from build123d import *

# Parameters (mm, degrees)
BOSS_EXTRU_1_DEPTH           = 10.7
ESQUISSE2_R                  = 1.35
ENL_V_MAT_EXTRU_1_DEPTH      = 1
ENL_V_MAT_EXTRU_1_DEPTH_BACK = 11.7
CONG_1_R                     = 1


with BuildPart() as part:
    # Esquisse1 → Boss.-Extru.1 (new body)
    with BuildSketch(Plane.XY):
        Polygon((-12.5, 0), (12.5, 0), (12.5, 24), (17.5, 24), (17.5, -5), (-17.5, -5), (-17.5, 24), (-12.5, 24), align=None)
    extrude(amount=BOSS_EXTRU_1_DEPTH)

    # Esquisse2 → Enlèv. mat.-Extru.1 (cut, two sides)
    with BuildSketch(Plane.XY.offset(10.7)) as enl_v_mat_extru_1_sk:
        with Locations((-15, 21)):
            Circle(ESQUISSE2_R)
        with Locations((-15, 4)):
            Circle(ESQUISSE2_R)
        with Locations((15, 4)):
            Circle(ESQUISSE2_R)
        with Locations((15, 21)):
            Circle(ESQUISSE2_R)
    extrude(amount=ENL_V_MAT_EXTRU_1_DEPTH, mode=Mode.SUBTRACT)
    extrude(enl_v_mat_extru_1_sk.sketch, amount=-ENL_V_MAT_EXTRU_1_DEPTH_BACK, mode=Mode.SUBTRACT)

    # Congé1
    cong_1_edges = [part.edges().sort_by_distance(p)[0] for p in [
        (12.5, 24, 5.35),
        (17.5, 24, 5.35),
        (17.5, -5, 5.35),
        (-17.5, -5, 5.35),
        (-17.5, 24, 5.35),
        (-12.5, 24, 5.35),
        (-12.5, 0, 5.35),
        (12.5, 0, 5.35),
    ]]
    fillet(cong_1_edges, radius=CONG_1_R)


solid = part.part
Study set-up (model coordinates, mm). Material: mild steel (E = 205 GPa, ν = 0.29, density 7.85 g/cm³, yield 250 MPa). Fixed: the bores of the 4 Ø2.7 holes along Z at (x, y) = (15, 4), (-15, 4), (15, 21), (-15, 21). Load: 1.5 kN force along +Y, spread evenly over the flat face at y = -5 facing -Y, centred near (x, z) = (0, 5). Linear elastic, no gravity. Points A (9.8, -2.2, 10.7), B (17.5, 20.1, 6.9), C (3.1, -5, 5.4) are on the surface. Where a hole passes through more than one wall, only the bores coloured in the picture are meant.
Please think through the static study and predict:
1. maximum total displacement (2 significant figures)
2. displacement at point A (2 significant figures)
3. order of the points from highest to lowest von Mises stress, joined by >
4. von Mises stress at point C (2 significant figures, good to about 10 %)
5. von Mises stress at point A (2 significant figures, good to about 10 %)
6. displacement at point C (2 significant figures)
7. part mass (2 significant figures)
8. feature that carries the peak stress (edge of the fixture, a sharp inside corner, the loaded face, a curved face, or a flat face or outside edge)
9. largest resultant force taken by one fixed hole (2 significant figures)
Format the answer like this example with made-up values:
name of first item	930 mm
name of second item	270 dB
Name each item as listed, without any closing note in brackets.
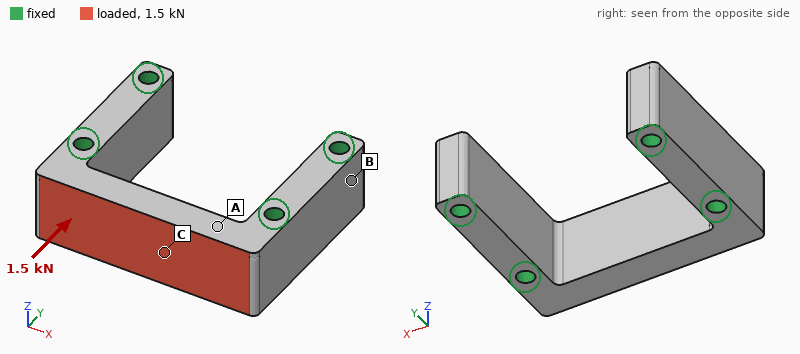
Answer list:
maximum total displacement	5.9 µm
displacement at point A	2.3 µm
order of the points from highest to lowest von Mises stress, joined by >	C > A > B
von Mises stress at point C	41 MPa
von Mises stress at point A	28 MPa
displacement at point C	5.2 µm
part mass	33 g
feature that carries the peak stress	a curved face
largest resultant force taken by one fixed hole	900 N
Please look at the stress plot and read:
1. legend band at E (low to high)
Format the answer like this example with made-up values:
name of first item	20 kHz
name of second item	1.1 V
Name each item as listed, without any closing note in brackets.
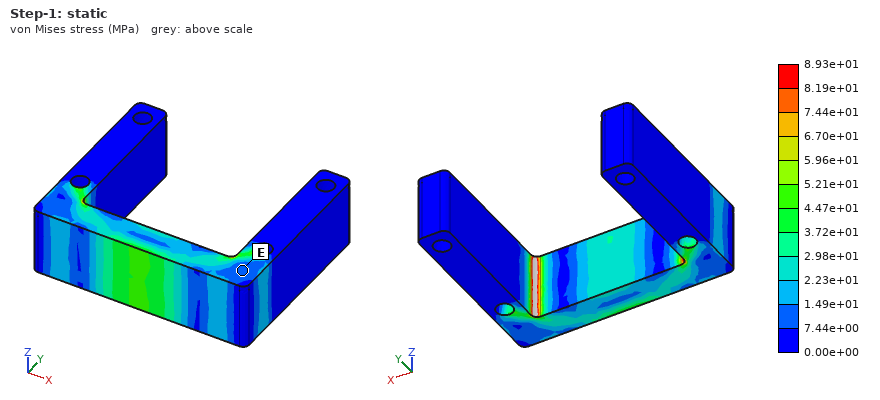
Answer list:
legend band at E	7.44e+00 to 1.49e+01 MPa
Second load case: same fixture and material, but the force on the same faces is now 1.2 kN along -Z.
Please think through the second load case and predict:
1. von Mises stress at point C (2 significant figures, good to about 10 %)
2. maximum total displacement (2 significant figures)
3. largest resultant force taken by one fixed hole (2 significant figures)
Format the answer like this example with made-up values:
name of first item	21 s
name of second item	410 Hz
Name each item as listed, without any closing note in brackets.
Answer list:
von Mises stress at point C	14 MPa
maximum total displacement	5.6 µm
largest resultant force taken by one fixed hole	610 N
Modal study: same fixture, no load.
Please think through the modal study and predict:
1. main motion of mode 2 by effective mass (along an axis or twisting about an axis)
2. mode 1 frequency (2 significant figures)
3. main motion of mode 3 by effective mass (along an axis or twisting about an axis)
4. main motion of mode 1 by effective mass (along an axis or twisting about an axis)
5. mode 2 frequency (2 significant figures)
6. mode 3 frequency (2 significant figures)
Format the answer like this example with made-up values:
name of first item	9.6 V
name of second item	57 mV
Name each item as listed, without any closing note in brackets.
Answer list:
main motion of mode 2 by effective mass	along Z
mode 1 frequency	24 kHz
main motion of mode 3 by effective mass	along X
main motion of mode 1 by effective mass	along Y
mode 2 frequency	27 kHz
mode 3 frequency	31 kHz
